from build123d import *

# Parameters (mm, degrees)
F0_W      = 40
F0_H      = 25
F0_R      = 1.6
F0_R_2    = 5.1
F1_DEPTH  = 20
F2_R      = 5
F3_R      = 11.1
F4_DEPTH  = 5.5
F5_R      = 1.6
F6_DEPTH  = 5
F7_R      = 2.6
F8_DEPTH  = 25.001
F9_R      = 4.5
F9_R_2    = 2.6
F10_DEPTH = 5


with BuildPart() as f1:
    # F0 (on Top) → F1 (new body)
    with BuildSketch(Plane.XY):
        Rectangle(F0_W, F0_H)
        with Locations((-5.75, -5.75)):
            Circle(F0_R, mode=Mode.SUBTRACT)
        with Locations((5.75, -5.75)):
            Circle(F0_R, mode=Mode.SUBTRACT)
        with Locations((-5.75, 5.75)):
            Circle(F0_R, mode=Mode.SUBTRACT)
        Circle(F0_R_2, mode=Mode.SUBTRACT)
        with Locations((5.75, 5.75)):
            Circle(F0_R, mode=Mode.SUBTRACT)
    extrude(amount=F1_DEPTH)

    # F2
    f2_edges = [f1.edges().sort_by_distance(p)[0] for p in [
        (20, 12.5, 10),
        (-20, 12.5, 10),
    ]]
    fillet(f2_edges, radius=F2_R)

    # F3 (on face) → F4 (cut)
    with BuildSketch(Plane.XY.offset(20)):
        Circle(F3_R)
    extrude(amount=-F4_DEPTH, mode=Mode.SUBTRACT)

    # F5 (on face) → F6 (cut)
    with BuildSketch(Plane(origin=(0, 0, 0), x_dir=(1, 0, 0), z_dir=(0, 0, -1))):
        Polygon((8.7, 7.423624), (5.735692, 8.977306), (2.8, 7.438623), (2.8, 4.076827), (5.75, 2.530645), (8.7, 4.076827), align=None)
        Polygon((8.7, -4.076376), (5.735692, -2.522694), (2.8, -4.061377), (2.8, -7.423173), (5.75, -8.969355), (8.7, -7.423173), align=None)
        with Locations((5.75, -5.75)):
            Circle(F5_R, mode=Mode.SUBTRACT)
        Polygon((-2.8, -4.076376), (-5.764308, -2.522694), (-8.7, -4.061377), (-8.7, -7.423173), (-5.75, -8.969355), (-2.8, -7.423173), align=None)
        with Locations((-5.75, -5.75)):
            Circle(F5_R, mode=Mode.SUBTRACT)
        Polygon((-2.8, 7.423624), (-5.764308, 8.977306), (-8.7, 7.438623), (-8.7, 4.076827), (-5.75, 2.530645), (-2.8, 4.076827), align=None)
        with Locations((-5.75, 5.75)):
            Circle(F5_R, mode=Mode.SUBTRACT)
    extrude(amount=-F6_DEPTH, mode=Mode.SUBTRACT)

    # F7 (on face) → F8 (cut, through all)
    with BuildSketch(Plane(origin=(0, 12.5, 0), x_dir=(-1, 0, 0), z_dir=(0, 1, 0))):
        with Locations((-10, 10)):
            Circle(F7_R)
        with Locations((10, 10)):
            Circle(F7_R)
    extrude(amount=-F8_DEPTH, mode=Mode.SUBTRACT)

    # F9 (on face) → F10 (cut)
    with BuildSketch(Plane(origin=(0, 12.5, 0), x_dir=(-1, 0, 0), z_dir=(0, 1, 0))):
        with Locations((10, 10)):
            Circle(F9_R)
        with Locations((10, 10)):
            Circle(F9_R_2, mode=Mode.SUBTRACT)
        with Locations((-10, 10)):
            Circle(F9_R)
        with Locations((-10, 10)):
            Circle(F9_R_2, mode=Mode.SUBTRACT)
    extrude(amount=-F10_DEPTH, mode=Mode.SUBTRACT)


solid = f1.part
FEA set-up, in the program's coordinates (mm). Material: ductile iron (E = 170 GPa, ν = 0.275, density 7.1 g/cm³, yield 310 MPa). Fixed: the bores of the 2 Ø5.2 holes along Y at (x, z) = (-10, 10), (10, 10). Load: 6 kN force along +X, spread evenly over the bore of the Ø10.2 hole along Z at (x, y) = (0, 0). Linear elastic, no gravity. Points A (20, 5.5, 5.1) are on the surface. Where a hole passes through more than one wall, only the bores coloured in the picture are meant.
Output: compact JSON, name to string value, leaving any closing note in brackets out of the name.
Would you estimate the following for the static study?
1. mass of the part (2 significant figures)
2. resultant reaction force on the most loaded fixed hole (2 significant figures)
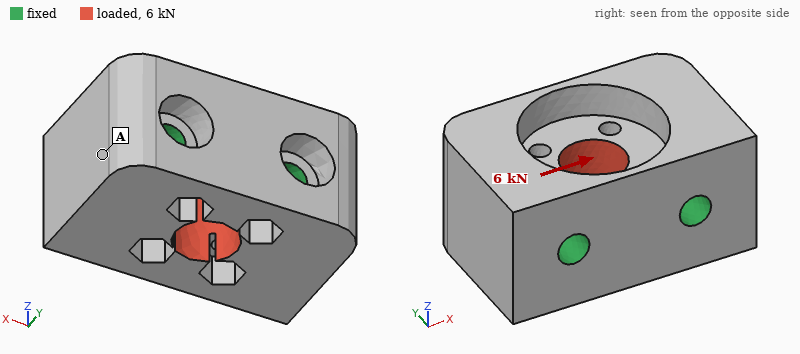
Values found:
{"mass of the part": "100 g", "resultant reaction force on the most loaded fixed hole": "3.0 kN"}
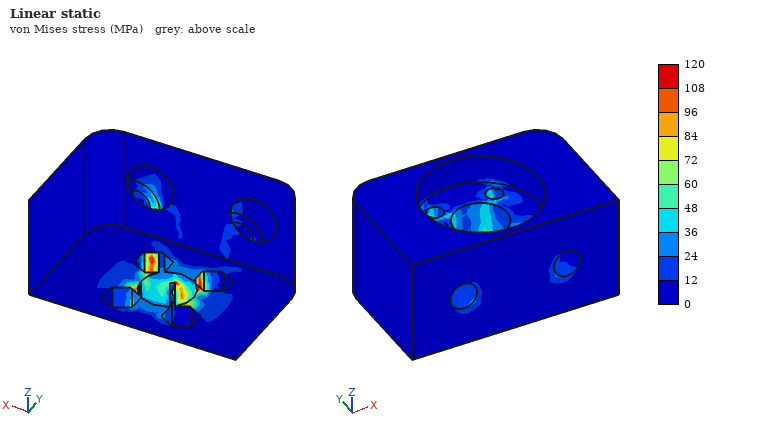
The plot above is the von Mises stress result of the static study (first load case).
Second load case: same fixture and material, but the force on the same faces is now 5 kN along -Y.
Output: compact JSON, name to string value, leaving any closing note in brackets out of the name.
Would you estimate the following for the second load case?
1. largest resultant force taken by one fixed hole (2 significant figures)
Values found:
{"largest resultant force taken by one fixed hole": "2.5 kN"}
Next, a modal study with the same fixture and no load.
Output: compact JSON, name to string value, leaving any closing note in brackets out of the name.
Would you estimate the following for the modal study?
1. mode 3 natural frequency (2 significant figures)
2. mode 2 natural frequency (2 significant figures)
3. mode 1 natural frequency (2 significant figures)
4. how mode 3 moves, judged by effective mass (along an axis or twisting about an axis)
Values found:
{"mode 3 natural frequency": "36 kHz", "mode 2 natural frequency": "34 kHz", "mode 1 natural frequency": "33 kHz", "how mode 3 moves, judged by effective mass": "along Z"}
